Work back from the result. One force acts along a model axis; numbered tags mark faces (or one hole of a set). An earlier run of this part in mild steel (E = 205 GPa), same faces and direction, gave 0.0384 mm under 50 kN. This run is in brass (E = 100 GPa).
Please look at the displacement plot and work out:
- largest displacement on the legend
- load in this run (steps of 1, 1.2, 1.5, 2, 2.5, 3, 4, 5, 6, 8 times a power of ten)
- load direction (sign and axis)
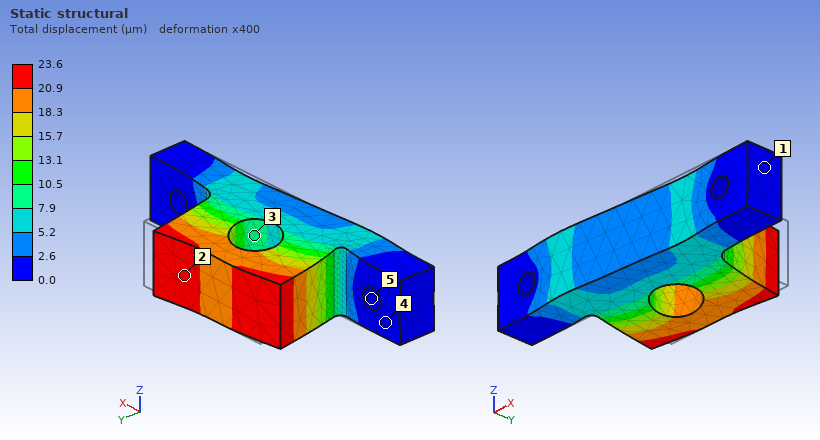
23.6 µm
15 kN
-X
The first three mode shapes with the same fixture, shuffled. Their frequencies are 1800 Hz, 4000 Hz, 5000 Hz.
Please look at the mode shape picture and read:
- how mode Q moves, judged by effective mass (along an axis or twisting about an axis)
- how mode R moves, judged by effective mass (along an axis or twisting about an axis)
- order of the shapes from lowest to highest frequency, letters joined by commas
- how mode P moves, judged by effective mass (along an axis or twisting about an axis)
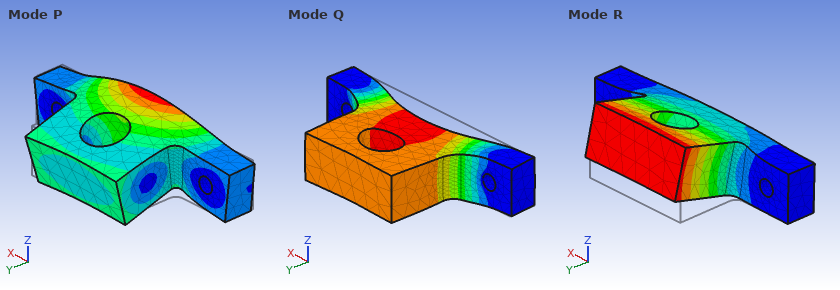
along Y
along Z
R, Q, P
along Z
